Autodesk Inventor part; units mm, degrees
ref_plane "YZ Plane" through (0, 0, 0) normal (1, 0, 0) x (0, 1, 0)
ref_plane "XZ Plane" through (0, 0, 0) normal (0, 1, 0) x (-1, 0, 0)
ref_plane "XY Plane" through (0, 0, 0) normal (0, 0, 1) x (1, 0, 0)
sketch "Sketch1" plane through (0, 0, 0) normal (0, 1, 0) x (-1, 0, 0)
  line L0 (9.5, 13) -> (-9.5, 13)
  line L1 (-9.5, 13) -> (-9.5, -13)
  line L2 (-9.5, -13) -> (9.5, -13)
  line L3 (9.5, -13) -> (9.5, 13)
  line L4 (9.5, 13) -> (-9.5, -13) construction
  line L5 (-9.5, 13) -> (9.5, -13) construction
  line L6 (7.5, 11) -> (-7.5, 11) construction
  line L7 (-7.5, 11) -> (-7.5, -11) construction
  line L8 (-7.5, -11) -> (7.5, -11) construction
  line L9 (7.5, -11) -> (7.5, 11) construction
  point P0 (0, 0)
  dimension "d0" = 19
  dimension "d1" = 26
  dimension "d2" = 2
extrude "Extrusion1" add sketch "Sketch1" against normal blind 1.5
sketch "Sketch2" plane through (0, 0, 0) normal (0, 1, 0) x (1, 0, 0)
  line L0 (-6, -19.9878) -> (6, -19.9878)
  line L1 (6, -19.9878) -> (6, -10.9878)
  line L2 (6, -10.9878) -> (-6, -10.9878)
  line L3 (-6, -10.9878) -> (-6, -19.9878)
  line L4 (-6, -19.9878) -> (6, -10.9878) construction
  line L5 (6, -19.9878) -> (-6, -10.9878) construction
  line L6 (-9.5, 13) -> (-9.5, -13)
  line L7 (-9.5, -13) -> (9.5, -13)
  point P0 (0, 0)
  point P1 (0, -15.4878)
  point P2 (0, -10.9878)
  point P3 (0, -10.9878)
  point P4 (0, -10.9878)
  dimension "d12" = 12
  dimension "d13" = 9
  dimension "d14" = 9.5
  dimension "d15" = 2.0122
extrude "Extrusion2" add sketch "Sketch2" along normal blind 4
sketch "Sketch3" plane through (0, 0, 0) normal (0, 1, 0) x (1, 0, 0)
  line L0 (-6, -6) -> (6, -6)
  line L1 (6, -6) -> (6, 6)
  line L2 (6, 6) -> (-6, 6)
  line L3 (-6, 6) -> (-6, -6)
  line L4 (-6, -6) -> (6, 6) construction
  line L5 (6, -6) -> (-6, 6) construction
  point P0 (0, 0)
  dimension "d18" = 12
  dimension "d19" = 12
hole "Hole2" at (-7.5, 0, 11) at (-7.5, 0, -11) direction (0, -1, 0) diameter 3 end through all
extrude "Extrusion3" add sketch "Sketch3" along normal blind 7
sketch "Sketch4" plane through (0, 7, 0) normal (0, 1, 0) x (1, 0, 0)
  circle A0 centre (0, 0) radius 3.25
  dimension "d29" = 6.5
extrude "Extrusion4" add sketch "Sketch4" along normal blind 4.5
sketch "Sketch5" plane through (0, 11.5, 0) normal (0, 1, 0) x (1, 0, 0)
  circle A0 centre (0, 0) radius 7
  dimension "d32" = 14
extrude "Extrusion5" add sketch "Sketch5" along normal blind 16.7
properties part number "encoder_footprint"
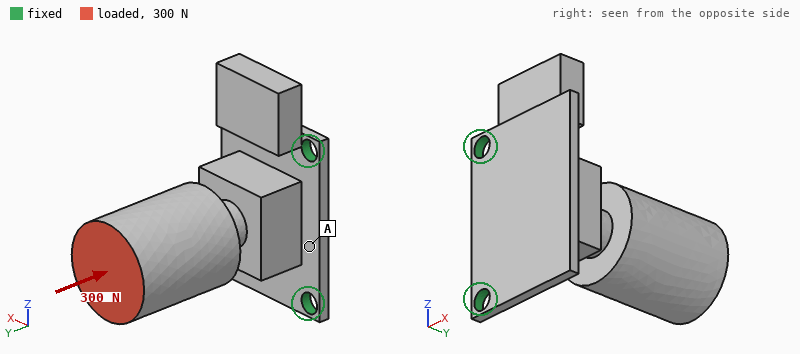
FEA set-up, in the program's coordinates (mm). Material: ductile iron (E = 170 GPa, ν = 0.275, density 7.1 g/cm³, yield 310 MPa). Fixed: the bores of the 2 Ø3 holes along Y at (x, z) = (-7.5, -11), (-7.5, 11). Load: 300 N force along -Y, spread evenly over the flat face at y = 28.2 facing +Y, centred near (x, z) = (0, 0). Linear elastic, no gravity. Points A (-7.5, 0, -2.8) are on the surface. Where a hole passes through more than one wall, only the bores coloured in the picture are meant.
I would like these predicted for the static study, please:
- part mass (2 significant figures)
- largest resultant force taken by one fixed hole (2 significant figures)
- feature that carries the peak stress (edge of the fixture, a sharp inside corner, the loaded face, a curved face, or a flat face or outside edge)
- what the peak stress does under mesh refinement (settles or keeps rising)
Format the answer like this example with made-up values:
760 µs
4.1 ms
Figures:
35 g
160 N
edge of the fixture
keeps rising
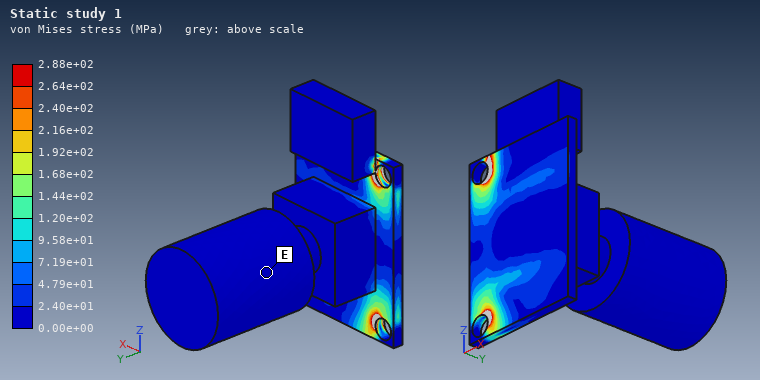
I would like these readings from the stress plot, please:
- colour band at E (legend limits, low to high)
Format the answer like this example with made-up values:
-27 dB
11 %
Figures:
0.00e+00 to 2.40e+01 MPa
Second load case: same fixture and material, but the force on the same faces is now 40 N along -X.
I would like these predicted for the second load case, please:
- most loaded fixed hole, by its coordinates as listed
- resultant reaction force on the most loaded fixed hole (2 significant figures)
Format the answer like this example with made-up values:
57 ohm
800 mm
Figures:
(-7.5, -11)
25 N
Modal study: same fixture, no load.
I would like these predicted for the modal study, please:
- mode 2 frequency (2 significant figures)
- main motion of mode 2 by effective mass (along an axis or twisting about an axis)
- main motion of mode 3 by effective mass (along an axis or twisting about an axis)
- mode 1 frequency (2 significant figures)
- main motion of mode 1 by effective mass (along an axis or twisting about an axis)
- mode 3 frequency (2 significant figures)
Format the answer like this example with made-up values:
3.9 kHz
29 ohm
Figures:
2300 Hz
along Z
along Y
890 Hz
along X
5300 Hz
